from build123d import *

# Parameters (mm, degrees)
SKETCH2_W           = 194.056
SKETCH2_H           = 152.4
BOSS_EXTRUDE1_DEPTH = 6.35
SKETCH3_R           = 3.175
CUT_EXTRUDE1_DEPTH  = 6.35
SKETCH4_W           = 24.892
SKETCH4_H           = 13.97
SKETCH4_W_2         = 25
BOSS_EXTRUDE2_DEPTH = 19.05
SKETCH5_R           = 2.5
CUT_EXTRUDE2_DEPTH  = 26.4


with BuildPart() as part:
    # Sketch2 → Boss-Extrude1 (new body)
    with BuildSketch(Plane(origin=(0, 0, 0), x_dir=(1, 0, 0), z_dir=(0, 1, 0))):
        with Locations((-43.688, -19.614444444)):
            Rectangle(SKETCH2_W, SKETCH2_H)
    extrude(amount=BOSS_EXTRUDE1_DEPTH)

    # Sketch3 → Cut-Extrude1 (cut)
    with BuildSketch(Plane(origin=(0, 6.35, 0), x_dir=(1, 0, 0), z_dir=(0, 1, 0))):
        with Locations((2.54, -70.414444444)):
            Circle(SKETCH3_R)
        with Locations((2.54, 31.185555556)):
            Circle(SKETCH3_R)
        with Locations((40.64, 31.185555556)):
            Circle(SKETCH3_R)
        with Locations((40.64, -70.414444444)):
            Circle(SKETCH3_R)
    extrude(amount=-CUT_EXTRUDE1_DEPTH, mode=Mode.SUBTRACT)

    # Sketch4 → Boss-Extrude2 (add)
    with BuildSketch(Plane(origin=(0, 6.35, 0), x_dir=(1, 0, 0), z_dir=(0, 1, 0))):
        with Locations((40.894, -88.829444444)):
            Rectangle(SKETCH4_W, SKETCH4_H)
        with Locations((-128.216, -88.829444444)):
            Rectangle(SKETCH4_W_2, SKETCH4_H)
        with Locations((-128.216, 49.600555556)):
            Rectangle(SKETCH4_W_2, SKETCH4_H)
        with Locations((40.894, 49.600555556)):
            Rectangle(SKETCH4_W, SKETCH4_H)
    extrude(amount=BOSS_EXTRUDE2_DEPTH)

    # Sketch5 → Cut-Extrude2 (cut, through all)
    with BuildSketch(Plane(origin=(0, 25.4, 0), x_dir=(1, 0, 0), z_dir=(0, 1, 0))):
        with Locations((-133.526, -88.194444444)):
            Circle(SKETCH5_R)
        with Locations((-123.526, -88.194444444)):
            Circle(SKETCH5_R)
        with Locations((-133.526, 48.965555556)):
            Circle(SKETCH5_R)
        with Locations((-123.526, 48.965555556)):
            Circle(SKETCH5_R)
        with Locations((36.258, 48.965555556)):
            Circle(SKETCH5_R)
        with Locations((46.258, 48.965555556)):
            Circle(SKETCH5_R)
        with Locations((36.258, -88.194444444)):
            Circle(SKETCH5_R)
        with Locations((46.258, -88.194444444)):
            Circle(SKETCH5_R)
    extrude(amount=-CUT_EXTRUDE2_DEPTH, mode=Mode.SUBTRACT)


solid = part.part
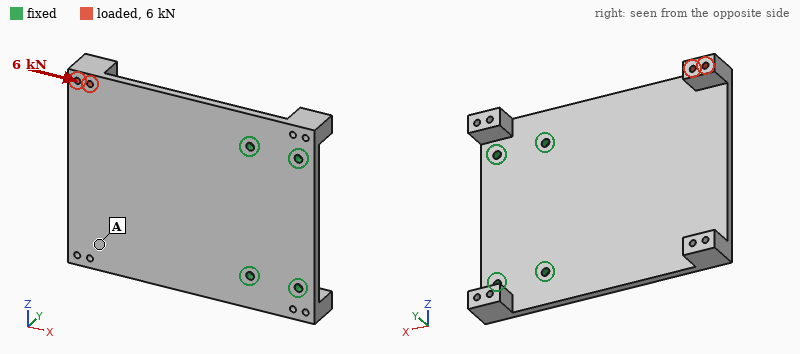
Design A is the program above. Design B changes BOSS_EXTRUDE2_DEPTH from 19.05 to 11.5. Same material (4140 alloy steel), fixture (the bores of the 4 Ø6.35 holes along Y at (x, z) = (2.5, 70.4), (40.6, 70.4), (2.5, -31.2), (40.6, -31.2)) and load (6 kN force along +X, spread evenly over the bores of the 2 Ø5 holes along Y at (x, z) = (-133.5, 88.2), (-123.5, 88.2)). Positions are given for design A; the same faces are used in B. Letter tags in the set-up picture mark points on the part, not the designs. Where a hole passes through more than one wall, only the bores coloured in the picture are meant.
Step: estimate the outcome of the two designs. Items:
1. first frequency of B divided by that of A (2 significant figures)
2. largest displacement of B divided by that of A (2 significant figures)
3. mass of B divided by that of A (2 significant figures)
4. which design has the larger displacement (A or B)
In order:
1.0
0.59
0.96
A
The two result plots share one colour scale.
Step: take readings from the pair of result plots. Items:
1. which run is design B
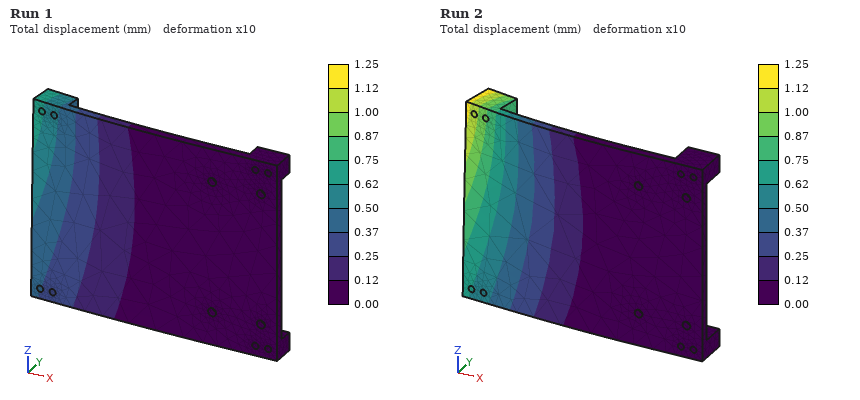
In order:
Run 1
